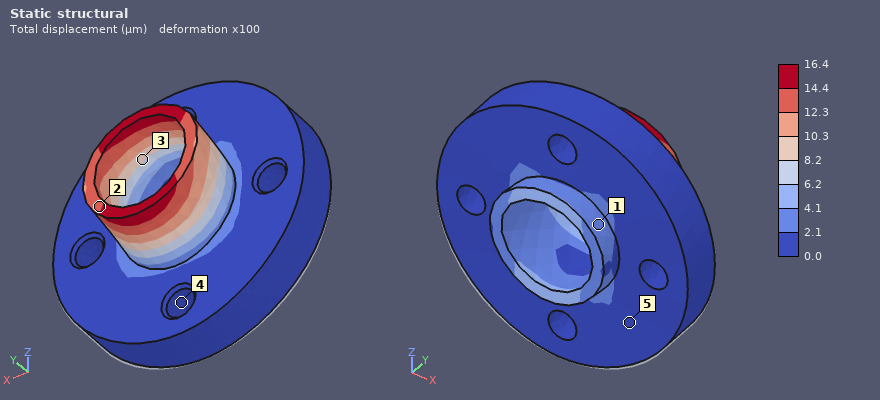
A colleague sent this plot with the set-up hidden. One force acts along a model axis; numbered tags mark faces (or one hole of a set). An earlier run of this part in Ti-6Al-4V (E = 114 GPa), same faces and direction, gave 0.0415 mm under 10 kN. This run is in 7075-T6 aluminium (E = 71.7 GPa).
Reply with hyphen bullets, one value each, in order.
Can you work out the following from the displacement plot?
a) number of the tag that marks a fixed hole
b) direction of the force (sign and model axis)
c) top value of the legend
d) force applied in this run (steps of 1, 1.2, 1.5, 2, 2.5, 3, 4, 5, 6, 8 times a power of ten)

- 4
- +Z
- 16.4 µm
- 2.5 kN
